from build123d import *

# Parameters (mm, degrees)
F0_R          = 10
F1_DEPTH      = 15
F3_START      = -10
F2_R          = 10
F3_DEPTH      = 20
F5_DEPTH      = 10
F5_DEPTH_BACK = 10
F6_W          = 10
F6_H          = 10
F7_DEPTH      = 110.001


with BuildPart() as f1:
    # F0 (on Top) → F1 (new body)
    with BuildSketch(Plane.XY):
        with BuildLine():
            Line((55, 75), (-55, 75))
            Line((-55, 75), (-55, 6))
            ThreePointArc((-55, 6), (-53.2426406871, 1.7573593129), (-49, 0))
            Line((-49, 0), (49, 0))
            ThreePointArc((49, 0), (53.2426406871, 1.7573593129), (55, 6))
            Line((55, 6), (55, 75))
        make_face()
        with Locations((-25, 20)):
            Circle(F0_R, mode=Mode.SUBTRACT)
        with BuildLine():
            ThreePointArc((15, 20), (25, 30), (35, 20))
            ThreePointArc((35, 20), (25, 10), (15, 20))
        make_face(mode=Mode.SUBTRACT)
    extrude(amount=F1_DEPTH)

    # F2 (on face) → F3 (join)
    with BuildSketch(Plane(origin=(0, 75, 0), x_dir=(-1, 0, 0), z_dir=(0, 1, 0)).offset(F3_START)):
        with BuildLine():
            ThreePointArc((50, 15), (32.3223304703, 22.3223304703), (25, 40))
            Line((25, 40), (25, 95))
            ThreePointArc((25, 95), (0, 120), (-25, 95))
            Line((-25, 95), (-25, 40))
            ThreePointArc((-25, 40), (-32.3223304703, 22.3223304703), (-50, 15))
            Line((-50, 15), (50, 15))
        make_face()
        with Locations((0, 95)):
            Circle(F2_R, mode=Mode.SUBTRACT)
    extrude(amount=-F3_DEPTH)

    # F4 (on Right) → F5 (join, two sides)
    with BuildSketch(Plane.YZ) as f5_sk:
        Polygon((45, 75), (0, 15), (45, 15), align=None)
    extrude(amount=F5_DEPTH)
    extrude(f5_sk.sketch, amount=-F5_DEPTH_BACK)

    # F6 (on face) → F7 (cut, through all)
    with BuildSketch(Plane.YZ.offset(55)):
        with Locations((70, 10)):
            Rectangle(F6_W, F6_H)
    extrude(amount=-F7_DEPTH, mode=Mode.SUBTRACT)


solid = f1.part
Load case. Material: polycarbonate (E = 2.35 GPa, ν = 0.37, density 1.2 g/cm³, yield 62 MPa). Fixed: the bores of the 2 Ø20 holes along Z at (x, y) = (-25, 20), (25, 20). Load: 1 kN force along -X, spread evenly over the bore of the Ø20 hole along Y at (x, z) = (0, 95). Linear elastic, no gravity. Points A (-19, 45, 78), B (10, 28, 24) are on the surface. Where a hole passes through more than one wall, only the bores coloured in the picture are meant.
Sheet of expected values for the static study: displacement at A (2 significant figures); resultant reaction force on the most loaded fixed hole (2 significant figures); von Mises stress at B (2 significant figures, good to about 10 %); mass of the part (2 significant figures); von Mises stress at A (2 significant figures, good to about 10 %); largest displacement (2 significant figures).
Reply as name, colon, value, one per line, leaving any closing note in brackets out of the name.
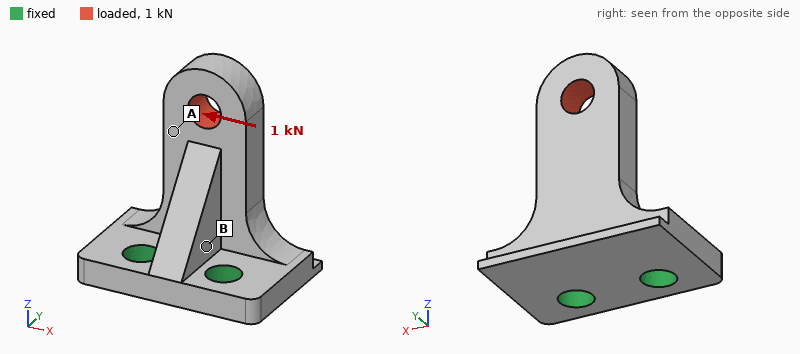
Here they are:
displacement at A: 0.62 mm
resultant reaction force on the most loaded fixed hole: 1.8 kN
von Mises stress at B: 5.0 MPa
mass of the part: 270 g
von Mises stress at A: 1.6 MPa
largest displacement: 1.1 mm
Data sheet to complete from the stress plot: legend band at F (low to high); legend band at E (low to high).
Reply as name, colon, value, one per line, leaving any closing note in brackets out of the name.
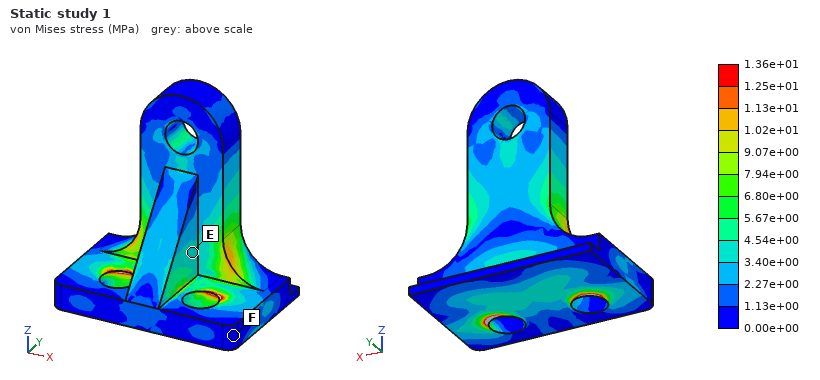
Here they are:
legend band at F: 0.00e+00 to 1.13e+00 MPa
legend band at E: 3.40e+00 to 4.54e+00 MPa
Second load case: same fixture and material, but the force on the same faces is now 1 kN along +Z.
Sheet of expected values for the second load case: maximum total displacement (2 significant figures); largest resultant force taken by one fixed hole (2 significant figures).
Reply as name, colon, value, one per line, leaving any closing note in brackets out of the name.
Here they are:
maximum total displacement: 0.42 mm
largest resultant force taken by one fixed hole: 510 N
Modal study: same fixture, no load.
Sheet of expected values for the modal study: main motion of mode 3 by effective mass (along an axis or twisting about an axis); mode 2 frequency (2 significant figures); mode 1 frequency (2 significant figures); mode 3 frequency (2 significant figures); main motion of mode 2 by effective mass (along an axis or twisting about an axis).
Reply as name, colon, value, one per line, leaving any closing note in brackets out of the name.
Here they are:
main motion of mode 3 by effective mass: along Z
mode 2 frequency: 720 Hz
mode 1 frequency: 550 Hz
mode 3 frequency: 1600 Hz
main motion of mode 2 by effective mass: along X
